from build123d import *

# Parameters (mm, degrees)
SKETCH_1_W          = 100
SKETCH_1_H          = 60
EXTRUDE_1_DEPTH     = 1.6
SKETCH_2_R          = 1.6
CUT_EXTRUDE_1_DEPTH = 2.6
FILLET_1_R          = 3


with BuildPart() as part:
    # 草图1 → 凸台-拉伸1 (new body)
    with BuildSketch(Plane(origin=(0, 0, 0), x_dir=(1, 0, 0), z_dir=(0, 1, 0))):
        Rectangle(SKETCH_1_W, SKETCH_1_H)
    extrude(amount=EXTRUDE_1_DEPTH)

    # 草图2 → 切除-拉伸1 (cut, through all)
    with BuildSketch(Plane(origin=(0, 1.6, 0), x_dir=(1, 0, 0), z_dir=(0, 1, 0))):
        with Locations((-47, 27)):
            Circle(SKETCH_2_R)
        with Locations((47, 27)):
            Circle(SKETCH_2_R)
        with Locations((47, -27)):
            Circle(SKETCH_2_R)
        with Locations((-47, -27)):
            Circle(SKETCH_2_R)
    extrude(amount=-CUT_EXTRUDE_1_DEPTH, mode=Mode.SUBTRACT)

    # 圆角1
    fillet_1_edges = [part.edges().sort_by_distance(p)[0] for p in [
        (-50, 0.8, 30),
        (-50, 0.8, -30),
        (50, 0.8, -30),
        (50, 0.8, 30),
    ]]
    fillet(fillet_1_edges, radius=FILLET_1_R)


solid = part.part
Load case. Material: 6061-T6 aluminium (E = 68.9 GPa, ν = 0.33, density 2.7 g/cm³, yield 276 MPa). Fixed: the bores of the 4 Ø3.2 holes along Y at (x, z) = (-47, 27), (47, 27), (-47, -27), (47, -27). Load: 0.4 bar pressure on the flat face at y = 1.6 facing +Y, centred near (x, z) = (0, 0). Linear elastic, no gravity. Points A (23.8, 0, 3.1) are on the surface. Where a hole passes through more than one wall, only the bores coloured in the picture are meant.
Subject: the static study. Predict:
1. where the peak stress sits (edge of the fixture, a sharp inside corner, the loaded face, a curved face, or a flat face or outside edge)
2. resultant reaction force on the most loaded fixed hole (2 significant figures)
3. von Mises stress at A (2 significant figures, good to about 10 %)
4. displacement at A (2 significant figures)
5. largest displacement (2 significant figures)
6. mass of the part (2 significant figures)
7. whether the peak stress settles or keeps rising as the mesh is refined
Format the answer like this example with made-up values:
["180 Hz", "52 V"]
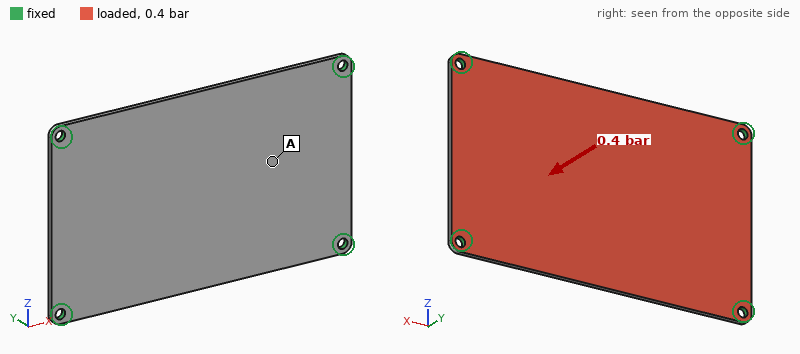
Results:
["edge of the fixture", "60 N", "20 MPa", "0.35 mm", "0.52 mm", "26 g", "keeps rising"]
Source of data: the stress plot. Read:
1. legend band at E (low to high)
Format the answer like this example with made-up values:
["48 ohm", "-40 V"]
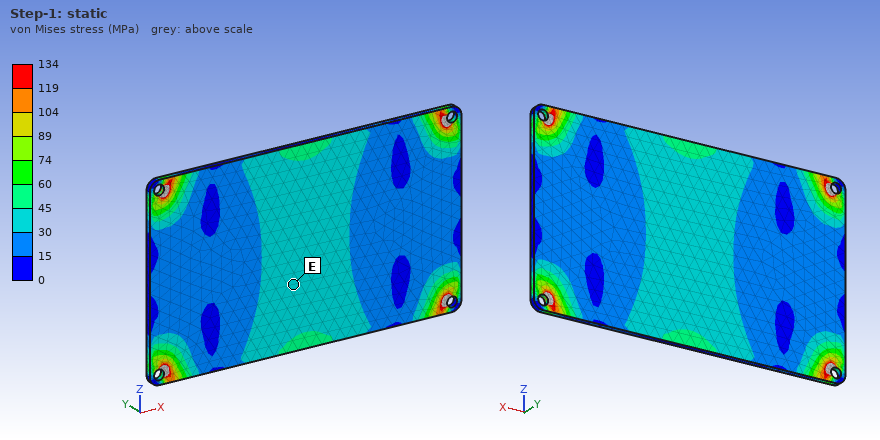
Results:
["30 to 45 MPa"]
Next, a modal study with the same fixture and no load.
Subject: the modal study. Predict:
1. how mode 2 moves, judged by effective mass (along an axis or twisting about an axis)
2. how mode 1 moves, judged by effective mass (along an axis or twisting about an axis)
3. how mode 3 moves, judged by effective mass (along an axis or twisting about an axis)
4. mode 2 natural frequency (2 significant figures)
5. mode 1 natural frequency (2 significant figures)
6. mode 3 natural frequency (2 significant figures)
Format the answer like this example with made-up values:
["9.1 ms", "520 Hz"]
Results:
["twisting about X", "along Y", "twisting about Z", "1400 Hz", "770 Hz", "2100 Hz"]
